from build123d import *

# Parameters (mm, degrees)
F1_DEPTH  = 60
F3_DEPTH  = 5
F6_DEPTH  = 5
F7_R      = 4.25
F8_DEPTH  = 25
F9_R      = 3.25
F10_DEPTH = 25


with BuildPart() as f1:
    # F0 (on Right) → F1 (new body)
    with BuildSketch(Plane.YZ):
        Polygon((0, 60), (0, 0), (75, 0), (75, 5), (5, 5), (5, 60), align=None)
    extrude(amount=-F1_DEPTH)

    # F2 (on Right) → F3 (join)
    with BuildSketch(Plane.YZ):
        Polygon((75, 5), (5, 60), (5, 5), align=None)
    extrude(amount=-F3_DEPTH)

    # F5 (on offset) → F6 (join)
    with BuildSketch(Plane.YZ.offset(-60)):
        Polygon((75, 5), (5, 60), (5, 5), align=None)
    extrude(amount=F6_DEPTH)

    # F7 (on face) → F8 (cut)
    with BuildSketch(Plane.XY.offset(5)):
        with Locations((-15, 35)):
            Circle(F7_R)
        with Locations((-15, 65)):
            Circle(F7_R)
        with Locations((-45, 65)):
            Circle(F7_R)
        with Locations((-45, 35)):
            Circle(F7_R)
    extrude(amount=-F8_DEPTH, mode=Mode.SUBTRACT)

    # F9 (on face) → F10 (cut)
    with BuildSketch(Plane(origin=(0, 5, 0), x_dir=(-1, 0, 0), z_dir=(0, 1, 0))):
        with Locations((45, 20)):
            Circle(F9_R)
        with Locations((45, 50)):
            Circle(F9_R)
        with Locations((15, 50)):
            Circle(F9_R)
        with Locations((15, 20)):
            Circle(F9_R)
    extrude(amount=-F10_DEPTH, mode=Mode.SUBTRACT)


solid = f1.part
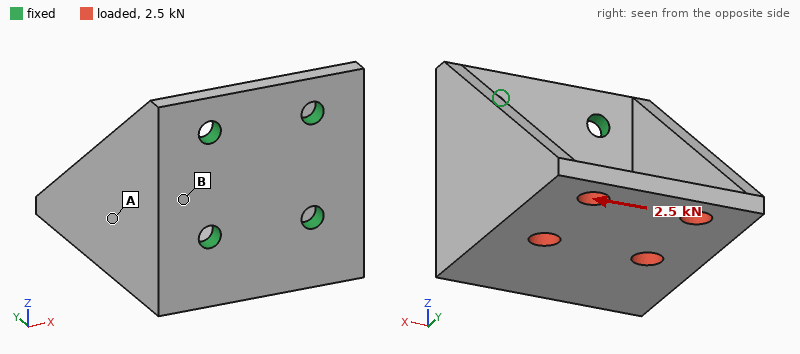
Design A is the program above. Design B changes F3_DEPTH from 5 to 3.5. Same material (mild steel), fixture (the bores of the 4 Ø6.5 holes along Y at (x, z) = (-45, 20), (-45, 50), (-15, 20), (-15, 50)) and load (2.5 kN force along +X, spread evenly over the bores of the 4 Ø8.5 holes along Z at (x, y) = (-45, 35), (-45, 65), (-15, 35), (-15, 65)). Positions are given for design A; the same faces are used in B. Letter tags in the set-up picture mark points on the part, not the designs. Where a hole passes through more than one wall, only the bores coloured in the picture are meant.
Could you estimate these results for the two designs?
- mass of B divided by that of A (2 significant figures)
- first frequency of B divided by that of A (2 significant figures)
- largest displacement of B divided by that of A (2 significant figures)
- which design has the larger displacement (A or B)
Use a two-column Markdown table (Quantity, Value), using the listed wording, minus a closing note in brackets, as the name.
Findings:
| Quantity | Value |
|---|---|
| mass of B divided by that of A | 0.95 |
| first frequency of B divided by that of A | 0.98 |
| largest displacement of B divided by that of A | 1.1 |
| which design has the larger displacement | B |
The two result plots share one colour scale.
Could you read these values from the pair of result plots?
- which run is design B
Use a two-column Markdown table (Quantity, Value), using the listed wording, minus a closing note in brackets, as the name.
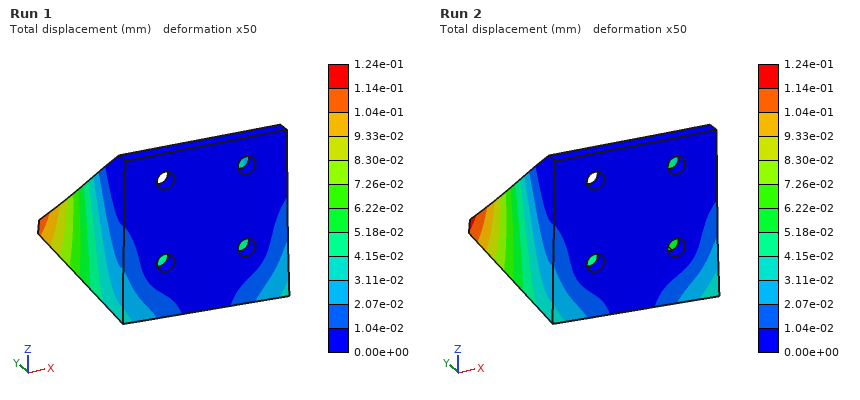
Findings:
| Quantity | Value |
|---|---|
| which run is design B | Run 2 |
